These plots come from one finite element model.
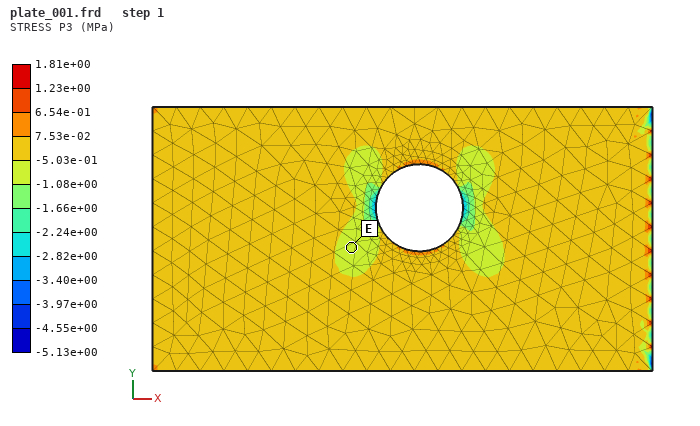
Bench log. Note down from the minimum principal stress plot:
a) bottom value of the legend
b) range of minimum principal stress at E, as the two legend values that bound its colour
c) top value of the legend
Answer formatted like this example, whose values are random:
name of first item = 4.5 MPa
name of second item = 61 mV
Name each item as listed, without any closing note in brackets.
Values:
bottom value of the legend = -5.13e+00 MPa
range of minimum principal stress at E, as the two legend values that bound its colour = -1.08e+00 to -5.03e-01 MPa
top value of the legend = 1.81e+00 MPa
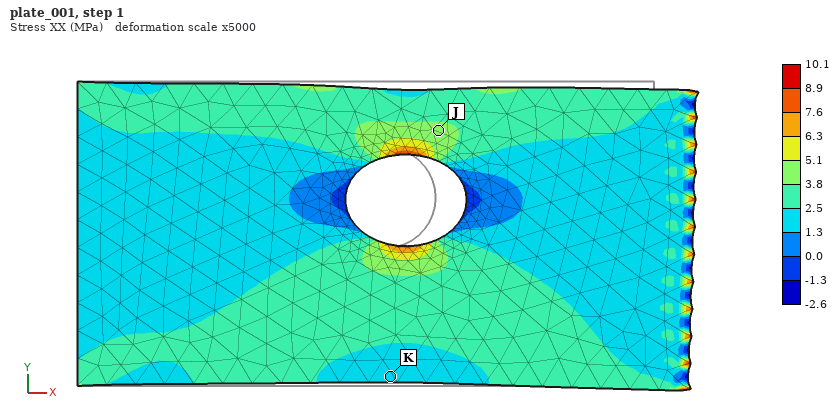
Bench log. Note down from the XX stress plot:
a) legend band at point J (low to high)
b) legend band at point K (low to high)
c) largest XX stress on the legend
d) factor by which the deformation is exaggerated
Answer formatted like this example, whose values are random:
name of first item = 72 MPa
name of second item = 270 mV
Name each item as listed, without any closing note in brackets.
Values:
legend band at point J = 3.8 to 5.1 MPa
legend band at point K = 1.3 to 2.5 MPa
largest XX stress on the legend = 10.1 MPa
factor by which the deformation is exaggerated = 5000
